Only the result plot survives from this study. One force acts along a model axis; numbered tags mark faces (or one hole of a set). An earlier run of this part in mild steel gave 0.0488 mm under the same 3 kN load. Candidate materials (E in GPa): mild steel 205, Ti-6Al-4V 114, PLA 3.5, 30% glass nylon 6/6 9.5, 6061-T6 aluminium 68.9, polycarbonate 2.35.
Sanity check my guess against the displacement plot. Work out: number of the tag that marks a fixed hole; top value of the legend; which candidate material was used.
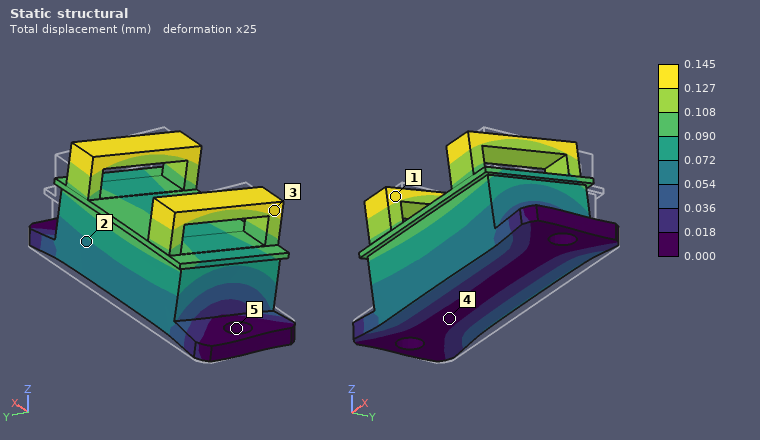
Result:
5
0.145 mm
6061-T6 aluminium
